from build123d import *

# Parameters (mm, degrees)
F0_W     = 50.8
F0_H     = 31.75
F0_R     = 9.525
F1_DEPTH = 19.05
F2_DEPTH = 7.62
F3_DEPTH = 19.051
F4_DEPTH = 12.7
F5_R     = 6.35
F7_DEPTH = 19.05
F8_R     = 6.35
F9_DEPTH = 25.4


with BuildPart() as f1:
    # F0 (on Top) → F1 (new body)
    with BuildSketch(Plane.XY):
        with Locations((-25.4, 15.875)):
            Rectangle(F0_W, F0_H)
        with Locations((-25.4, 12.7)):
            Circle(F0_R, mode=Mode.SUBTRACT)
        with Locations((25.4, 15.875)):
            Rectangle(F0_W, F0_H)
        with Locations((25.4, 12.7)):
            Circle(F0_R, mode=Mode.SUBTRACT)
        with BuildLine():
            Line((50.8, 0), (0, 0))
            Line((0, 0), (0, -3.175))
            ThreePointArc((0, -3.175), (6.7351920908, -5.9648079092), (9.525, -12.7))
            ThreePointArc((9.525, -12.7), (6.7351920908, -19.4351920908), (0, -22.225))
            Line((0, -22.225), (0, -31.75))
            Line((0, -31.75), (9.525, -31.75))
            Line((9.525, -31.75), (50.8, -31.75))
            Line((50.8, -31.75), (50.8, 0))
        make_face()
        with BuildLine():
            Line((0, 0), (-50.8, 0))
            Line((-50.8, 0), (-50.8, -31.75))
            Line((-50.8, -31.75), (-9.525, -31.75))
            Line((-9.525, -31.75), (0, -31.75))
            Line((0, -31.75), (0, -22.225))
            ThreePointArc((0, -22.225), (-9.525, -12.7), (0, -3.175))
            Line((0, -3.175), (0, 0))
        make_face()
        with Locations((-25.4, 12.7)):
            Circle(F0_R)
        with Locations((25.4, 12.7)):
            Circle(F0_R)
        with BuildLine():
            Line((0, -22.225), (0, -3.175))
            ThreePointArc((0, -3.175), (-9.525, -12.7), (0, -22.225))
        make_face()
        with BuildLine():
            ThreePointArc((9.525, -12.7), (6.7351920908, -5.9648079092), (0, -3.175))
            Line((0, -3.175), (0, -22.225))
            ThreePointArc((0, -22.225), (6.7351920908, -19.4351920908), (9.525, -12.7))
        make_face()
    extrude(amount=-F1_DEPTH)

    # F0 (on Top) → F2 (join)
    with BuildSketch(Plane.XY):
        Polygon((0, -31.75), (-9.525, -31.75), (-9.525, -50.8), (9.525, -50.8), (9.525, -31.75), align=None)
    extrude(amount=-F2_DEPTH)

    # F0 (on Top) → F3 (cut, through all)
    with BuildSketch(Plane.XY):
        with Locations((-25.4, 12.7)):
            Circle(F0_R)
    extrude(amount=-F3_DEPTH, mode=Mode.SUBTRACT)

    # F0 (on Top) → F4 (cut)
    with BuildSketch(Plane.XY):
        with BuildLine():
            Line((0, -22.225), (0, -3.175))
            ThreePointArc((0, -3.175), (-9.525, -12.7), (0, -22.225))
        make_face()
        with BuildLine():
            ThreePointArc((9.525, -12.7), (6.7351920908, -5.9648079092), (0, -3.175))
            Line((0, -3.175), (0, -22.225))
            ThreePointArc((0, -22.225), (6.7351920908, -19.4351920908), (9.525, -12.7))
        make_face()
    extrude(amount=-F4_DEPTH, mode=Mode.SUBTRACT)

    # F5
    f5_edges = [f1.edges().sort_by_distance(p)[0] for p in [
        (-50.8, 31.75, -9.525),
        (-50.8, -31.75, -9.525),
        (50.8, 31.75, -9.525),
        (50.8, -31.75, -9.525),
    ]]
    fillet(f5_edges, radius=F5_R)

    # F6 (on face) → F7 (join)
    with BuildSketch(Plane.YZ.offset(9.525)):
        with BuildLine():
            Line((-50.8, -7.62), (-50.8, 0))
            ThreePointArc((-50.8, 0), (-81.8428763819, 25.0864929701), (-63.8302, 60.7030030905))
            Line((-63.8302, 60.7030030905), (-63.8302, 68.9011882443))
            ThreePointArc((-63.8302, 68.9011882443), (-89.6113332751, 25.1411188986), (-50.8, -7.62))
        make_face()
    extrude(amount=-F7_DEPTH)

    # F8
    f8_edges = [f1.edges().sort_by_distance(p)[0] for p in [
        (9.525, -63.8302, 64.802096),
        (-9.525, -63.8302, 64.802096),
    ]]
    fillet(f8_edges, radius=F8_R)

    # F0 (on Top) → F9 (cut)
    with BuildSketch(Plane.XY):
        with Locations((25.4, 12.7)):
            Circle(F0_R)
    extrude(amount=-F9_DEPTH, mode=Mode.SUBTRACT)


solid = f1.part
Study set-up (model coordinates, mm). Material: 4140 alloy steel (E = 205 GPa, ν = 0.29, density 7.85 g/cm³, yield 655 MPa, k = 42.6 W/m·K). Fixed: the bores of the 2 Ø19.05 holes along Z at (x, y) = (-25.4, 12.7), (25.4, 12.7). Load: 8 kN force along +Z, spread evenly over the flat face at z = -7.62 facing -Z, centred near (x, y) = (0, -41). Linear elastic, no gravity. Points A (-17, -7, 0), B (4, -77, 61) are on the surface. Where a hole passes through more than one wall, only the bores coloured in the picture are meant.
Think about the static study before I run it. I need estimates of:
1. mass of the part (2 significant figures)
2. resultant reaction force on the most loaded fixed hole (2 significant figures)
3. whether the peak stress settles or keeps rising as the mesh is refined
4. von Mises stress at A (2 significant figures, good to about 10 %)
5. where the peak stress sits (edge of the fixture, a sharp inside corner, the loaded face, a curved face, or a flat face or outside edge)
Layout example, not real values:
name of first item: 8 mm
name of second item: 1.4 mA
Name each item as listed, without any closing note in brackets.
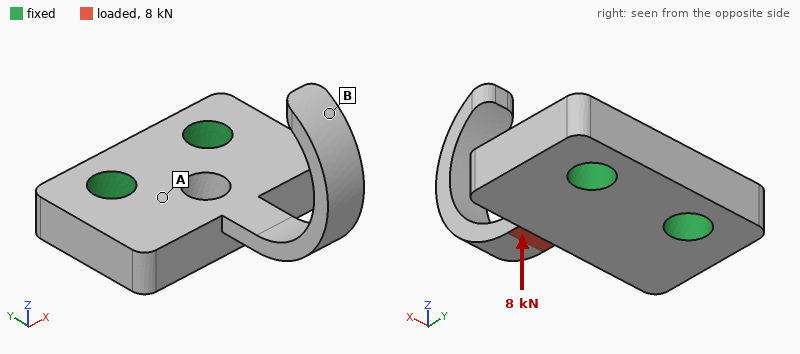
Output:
mass of the part: 980 g
resultant reaction force on the most loaded fixed hole: 4.0 kN
whether the peak stress settles or keeps rising as the mesh is refined: keeps rising
von Mises stress at A: 75 MPa
where the peak stress sits: a sharp inside corner
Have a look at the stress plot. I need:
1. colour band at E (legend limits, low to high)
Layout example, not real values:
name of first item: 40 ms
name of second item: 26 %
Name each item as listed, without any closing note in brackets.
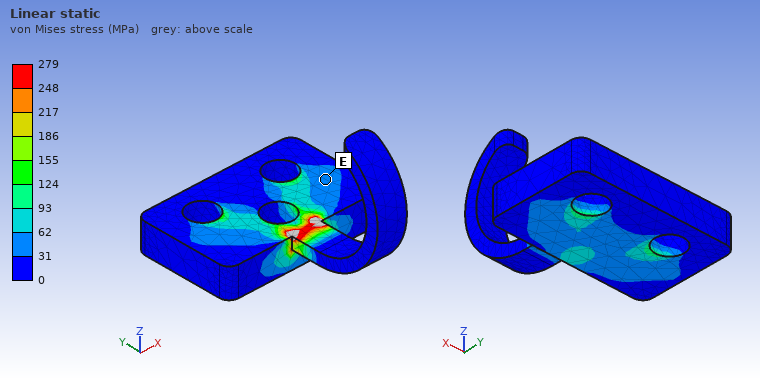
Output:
colour band at E: 31 to 62 MPa
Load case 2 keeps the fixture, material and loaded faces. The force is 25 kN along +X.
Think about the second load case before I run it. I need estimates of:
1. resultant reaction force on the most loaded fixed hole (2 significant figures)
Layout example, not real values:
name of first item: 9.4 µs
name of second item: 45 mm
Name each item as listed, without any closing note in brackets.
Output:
resultant reaction force on the most loaded fixed hole: 23 kN
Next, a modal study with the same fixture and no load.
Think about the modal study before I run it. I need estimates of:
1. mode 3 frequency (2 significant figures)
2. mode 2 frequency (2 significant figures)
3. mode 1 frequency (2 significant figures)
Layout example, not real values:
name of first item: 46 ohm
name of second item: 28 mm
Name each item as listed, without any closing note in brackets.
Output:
mode 3 frequency: 1600 Hz
mode 2 frequency: 750 Hz
mode 1 frequency: 530 Hz
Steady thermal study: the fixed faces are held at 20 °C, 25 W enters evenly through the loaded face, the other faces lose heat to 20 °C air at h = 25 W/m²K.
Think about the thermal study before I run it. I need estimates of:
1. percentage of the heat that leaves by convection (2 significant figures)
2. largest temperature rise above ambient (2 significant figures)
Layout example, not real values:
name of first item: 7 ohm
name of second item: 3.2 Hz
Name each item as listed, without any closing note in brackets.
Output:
percentage of the heat that leaves by convection: 27 %
largest temperature rise above ambient: 58 K
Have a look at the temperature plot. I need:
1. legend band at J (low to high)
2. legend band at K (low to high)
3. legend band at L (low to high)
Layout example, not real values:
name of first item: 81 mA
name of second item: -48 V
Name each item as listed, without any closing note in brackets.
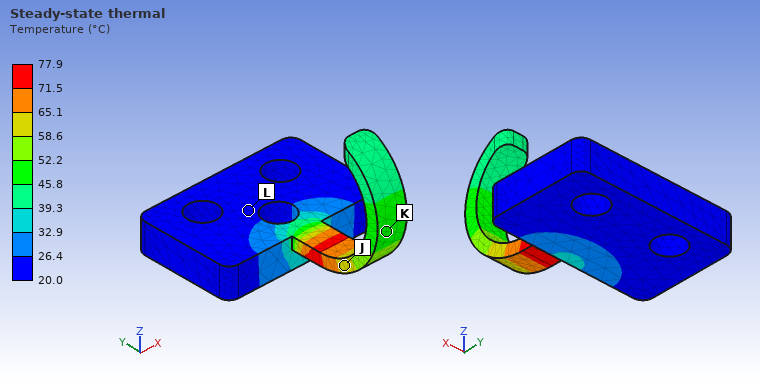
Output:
legend band at J: 58.6 to 65.1 °C
legend band at K: 45.8 to 52.2 °C
legend band at L: 20.0 to 26.4 °C
